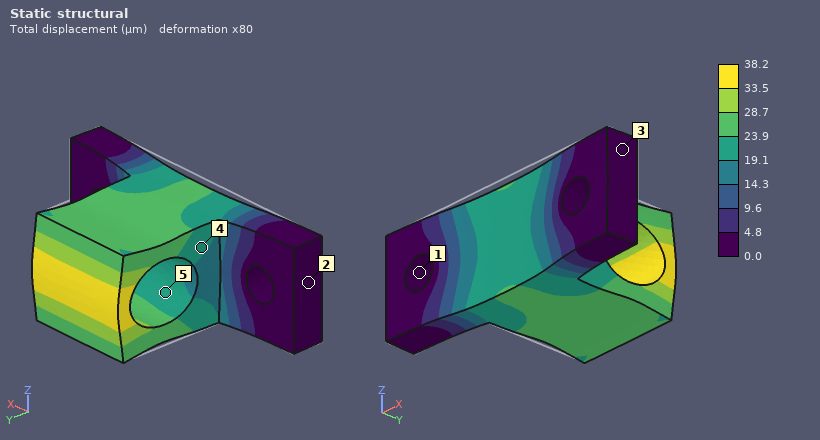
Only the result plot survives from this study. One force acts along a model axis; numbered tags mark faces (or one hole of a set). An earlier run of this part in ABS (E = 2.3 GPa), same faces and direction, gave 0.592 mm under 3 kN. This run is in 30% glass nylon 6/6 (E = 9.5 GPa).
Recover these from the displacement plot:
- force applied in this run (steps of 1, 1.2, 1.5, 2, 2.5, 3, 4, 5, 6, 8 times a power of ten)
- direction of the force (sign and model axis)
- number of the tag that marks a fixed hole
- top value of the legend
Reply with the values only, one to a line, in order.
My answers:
800 N
+Y
1
38.2 µm
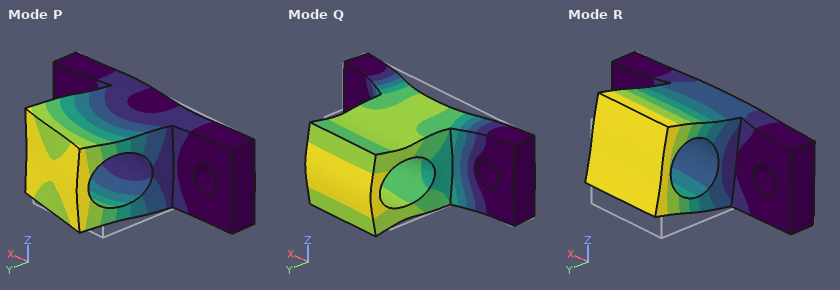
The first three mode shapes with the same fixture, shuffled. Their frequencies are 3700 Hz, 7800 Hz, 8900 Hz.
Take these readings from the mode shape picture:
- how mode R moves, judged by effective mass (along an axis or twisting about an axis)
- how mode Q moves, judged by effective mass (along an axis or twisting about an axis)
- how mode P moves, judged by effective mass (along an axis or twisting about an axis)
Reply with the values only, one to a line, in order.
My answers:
along Z
along Y
along X
